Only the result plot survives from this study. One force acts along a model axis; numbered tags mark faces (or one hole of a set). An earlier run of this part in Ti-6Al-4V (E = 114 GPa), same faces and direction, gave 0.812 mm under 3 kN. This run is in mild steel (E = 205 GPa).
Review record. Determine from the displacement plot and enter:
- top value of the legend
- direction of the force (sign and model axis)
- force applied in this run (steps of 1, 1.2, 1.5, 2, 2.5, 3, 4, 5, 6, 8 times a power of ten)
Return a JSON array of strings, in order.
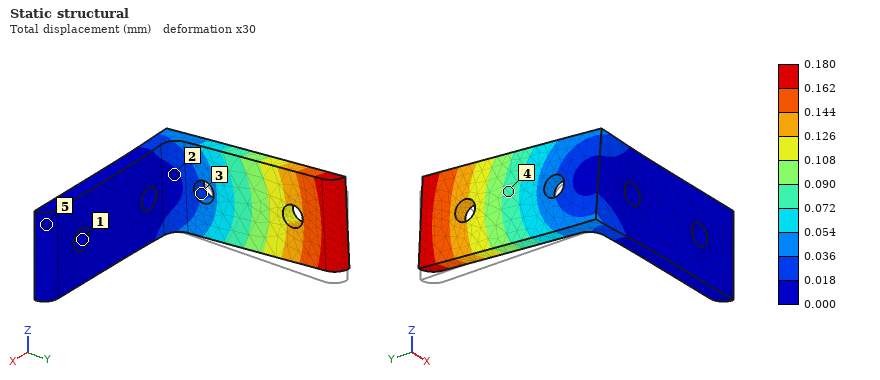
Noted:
["0.180 mm", "+Z", "1.2 kN"]
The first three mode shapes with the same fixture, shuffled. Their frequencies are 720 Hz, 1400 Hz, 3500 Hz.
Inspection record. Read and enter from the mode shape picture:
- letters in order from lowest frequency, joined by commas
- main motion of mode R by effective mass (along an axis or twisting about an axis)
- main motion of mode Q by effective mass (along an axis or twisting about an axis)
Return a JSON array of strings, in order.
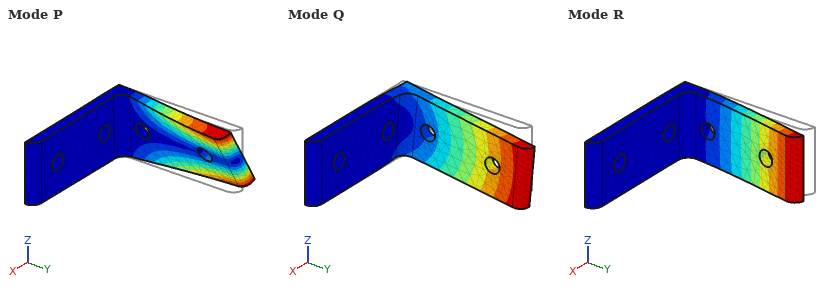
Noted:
["R, Q, P", "along X", "along Z"]
